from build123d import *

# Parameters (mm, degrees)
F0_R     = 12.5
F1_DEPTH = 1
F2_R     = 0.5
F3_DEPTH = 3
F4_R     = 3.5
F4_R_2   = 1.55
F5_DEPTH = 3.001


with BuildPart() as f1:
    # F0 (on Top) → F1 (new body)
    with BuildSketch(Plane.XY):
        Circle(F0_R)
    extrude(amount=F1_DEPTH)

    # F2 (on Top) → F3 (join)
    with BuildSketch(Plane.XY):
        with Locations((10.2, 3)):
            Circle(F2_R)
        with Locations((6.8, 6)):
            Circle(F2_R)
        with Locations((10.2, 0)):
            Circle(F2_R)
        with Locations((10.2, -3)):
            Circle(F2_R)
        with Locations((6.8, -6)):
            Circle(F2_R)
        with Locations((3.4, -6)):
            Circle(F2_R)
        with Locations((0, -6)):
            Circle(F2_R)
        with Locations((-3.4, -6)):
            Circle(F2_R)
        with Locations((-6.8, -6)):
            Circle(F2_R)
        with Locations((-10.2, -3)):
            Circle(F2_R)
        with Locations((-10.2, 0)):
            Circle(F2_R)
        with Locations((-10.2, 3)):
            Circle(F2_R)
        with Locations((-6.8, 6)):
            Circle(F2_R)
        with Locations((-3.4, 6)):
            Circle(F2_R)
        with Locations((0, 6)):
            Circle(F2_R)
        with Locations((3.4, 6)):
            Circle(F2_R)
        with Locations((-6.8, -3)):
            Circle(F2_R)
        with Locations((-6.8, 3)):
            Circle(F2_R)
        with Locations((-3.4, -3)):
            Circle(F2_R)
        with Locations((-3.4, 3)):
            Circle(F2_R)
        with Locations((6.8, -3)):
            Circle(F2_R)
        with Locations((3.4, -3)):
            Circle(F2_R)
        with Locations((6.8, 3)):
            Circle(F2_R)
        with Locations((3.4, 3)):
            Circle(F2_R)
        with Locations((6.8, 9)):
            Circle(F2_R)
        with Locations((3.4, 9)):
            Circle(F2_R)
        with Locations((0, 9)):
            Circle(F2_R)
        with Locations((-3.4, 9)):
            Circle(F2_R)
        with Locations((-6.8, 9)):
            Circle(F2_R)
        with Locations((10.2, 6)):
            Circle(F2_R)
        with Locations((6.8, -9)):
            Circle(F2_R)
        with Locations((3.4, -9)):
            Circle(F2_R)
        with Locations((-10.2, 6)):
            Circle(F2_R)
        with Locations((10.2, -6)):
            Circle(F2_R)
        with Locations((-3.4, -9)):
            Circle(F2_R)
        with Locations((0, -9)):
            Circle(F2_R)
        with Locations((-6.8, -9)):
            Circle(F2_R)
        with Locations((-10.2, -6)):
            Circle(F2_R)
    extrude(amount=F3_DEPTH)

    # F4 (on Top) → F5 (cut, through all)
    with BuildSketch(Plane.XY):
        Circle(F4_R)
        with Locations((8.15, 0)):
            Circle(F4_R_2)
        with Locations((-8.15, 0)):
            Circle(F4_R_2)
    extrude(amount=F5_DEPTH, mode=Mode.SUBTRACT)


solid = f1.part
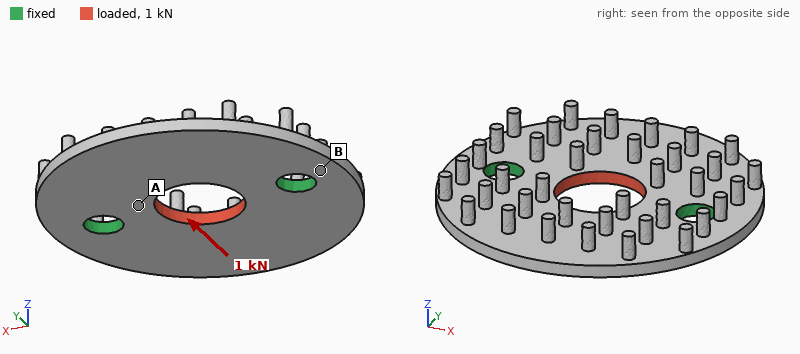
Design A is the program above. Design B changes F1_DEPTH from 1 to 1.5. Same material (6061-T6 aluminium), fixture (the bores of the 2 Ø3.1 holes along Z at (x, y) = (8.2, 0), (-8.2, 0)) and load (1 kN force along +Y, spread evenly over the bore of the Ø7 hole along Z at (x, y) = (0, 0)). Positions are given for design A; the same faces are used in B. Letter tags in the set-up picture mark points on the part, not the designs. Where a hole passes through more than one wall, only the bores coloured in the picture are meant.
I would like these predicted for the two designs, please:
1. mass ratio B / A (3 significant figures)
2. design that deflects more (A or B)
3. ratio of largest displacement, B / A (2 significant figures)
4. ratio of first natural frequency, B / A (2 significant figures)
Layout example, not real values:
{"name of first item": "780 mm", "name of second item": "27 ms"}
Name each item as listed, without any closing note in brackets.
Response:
{"mass ratio B / A": "1.41", "design that deflects more": "A", "ratio of largest displacement, B / A": "0.67", "ratio of first natural frequency, B / A": "1.5"}
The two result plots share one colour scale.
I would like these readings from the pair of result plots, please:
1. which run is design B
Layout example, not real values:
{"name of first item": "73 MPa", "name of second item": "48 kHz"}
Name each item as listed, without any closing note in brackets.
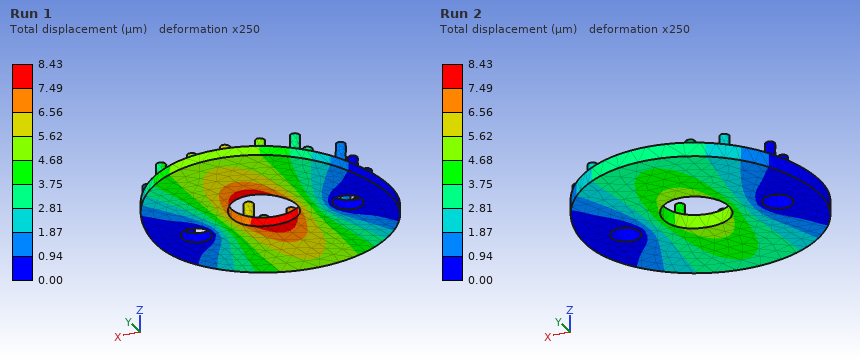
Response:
{"which run is design B": "Run 2"}
